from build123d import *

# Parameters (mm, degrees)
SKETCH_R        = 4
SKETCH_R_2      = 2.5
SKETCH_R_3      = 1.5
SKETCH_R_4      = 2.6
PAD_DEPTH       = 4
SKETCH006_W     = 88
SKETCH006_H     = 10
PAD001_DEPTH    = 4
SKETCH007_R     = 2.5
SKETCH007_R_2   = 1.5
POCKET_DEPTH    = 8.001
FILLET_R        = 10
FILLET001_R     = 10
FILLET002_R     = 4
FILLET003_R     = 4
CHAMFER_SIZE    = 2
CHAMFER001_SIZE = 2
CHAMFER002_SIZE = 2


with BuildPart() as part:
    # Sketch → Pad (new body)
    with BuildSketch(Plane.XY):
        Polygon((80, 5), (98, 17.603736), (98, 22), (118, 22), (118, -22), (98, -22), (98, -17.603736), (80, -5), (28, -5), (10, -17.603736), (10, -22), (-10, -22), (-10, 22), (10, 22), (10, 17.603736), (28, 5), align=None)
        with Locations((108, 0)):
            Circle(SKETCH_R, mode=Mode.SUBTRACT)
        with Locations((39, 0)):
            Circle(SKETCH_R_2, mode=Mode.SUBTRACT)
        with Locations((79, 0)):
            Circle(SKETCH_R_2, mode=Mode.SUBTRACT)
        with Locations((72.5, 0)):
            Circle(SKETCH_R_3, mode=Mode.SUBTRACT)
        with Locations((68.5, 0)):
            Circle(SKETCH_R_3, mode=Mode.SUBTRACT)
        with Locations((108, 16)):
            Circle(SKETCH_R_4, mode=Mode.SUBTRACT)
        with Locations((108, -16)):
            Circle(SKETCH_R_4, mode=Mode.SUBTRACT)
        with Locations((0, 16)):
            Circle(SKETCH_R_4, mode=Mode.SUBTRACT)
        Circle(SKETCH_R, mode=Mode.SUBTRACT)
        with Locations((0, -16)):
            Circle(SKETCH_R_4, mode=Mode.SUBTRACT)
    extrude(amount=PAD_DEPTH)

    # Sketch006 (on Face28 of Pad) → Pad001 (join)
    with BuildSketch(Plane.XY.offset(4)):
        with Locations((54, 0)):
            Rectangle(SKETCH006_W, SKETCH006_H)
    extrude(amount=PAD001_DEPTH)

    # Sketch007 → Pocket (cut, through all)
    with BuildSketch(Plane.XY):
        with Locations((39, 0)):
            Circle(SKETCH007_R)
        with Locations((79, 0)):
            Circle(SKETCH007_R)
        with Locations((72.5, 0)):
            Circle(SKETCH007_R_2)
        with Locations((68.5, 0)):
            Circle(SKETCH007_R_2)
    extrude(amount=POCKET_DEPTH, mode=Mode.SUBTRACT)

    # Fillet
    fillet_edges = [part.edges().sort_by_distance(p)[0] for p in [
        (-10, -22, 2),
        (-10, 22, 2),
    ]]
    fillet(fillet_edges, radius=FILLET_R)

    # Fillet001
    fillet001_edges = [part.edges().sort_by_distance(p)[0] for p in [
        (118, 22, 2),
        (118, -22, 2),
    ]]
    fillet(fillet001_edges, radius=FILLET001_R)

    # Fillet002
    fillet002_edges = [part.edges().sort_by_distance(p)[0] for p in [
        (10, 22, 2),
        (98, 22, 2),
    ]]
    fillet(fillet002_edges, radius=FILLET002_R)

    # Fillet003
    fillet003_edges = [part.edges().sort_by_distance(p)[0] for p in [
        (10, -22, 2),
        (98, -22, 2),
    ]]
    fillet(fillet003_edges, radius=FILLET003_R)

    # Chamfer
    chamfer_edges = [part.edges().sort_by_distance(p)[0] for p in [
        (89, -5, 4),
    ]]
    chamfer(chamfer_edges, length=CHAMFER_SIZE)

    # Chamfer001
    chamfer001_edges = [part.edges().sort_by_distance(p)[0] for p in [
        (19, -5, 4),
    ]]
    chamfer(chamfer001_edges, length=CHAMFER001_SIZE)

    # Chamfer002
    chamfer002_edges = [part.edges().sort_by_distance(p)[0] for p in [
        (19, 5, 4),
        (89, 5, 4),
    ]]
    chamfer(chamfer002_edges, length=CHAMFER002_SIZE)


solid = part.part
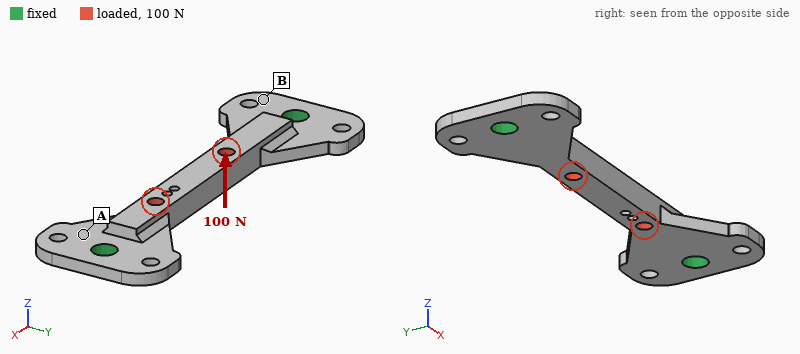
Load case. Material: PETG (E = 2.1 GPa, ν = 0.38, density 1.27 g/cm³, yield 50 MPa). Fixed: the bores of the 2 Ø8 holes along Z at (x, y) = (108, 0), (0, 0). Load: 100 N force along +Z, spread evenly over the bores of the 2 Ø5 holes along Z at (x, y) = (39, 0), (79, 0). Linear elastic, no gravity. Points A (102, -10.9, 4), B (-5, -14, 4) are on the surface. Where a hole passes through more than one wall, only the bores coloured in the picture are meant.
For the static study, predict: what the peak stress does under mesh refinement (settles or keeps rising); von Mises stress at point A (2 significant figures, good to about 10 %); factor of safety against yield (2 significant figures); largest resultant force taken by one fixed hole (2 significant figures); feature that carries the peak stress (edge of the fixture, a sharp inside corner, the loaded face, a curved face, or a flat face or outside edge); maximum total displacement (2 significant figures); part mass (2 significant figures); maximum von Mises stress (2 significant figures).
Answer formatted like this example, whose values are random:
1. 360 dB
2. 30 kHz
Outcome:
1. settles
2. 4.0 MPa
3. 2.3
4. 120 N
5. the loaded face
6. 0.66 mm
7. 18 g
8. 22 MPa
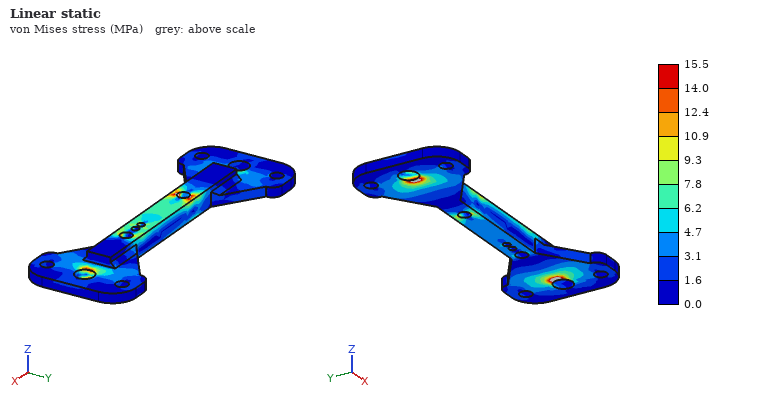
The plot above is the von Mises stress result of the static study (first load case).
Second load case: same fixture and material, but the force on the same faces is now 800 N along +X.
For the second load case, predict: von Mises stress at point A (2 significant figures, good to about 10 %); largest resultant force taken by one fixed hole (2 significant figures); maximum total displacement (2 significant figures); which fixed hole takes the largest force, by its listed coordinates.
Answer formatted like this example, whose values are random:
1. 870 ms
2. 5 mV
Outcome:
1. 2.9 MPa
2. 430 N
3. 0.15 mm
4. (108, 0)
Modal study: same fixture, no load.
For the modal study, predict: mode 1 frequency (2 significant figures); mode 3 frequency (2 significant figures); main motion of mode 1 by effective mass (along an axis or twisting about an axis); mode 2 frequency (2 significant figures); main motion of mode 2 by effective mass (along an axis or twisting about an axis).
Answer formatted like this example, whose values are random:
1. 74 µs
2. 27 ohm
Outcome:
1. 800 Hz
2. 1900 Hz
3. along Z
4. 1500 Hz
5. along Y
